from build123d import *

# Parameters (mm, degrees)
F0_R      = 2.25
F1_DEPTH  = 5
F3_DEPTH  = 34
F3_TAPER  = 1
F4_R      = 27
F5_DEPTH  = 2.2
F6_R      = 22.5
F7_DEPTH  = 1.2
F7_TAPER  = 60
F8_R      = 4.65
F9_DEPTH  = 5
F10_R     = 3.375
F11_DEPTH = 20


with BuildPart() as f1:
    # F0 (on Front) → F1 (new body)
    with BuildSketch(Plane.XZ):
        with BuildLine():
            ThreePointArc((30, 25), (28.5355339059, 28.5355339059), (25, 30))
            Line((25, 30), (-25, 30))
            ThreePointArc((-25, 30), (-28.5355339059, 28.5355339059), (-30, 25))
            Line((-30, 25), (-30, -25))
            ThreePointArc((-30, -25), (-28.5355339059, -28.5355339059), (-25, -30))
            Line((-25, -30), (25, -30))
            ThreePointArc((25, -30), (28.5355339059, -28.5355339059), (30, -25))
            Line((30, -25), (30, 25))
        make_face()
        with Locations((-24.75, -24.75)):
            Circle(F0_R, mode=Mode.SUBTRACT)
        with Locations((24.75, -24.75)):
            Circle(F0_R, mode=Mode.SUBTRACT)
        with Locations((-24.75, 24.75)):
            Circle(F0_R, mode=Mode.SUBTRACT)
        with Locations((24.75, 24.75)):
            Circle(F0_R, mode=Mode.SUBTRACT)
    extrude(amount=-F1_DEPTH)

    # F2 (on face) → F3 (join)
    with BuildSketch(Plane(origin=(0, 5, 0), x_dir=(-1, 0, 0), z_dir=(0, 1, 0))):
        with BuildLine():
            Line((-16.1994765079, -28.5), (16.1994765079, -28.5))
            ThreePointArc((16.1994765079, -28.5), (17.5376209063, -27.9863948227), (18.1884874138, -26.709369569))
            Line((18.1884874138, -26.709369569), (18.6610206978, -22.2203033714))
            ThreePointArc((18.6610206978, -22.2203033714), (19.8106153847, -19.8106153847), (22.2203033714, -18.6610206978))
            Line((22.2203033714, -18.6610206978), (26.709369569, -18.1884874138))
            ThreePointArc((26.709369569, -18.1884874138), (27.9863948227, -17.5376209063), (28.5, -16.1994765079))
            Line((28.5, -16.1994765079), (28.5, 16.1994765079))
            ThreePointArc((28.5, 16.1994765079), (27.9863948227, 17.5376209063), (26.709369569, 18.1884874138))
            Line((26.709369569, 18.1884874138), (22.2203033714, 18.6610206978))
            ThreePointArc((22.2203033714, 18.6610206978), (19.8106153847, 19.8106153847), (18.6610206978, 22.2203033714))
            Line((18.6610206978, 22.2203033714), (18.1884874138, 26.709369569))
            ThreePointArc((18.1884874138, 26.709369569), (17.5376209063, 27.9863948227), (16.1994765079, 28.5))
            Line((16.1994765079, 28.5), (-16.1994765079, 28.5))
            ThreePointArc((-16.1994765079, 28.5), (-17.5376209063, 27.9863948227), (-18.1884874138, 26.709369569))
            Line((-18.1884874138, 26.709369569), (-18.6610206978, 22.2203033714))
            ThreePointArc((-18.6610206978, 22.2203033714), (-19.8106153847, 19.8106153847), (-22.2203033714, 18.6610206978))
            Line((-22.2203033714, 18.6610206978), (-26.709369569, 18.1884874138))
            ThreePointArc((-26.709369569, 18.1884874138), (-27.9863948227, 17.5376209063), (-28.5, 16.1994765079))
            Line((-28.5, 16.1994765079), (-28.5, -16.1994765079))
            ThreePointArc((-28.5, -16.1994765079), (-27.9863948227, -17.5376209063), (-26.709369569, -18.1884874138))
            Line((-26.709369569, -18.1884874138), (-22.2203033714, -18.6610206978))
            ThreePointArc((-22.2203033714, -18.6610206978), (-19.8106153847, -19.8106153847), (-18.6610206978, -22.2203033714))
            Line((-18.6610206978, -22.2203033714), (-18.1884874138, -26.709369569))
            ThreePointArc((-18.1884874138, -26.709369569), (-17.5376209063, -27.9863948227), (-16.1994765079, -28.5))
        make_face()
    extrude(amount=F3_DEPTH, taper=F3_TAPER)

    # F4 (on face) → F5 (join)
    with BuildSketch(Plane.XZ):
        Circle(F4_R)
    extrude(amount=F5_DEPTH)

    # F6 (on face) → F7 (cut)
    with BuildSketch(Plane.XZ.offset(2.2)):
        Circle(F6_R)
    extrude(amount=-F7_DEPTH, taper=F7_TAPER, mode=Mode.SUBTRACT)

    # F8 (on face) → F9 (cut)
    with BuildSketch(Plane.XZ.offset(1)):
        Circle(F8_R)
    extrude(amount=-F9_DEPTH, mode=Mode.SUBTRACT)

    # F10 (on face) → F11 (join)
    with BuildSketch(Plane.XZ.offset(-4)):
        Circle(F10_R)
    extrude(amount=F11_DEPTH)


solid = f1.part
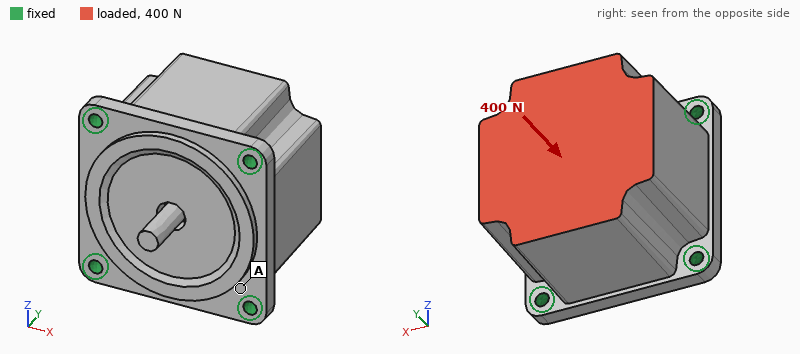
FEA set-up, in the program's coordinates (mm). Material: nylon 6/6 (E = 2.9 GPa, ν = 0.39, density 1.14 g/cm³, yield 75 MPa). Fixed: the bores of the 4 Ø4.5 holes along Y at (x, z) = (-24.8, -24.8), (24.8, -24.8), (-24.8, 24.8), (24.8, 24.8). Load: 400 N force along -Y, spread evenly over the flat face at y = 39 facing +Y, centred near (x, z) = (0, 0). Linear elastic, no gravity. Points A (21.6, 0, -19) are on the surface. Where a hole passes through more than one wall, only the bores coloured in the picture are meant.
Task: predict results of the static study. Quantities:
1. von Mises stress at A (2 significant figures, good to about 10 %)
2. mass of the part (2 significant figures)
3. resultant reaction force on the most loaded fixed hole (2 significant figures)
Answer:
0.91 MPa
130 g
110 N
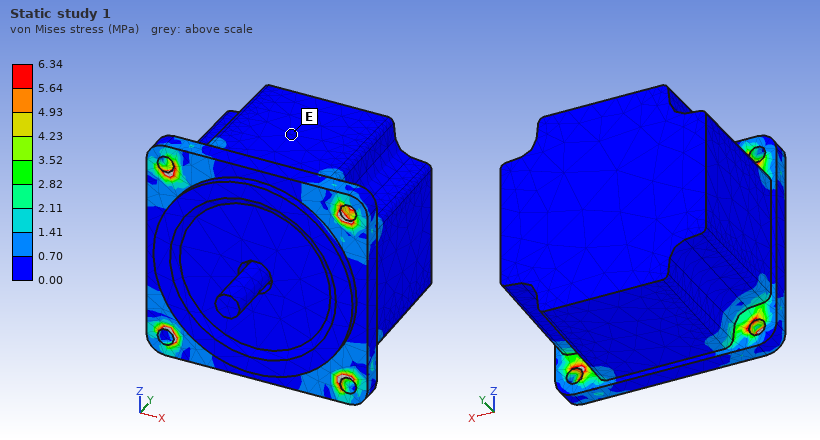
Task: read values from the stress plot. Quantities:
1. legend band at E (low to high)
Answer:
0.00 to 0.70 MPa
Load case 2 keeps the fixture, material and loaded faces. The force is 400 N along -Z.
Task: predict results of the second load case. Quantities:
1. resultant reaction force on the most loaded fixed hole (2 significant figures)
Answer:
200 N
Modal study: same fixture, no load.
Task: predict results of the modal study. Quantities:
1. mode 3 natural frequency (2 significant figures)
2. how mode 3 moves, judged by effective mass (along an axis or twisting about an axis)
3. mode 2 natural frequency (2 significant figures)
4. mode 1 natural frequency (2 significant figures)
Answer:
2200 Hz
along Y
1900 Hz
1900 Hz
